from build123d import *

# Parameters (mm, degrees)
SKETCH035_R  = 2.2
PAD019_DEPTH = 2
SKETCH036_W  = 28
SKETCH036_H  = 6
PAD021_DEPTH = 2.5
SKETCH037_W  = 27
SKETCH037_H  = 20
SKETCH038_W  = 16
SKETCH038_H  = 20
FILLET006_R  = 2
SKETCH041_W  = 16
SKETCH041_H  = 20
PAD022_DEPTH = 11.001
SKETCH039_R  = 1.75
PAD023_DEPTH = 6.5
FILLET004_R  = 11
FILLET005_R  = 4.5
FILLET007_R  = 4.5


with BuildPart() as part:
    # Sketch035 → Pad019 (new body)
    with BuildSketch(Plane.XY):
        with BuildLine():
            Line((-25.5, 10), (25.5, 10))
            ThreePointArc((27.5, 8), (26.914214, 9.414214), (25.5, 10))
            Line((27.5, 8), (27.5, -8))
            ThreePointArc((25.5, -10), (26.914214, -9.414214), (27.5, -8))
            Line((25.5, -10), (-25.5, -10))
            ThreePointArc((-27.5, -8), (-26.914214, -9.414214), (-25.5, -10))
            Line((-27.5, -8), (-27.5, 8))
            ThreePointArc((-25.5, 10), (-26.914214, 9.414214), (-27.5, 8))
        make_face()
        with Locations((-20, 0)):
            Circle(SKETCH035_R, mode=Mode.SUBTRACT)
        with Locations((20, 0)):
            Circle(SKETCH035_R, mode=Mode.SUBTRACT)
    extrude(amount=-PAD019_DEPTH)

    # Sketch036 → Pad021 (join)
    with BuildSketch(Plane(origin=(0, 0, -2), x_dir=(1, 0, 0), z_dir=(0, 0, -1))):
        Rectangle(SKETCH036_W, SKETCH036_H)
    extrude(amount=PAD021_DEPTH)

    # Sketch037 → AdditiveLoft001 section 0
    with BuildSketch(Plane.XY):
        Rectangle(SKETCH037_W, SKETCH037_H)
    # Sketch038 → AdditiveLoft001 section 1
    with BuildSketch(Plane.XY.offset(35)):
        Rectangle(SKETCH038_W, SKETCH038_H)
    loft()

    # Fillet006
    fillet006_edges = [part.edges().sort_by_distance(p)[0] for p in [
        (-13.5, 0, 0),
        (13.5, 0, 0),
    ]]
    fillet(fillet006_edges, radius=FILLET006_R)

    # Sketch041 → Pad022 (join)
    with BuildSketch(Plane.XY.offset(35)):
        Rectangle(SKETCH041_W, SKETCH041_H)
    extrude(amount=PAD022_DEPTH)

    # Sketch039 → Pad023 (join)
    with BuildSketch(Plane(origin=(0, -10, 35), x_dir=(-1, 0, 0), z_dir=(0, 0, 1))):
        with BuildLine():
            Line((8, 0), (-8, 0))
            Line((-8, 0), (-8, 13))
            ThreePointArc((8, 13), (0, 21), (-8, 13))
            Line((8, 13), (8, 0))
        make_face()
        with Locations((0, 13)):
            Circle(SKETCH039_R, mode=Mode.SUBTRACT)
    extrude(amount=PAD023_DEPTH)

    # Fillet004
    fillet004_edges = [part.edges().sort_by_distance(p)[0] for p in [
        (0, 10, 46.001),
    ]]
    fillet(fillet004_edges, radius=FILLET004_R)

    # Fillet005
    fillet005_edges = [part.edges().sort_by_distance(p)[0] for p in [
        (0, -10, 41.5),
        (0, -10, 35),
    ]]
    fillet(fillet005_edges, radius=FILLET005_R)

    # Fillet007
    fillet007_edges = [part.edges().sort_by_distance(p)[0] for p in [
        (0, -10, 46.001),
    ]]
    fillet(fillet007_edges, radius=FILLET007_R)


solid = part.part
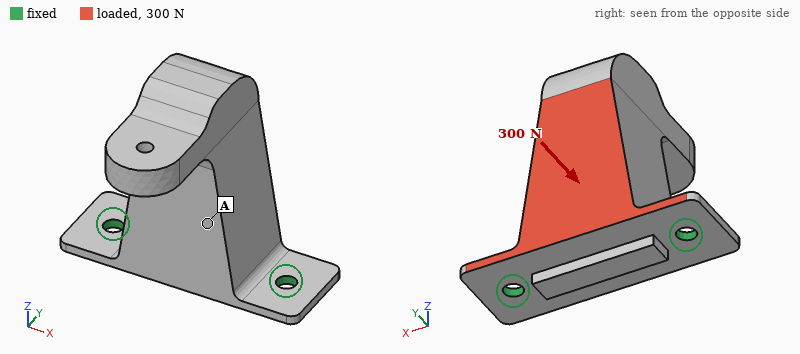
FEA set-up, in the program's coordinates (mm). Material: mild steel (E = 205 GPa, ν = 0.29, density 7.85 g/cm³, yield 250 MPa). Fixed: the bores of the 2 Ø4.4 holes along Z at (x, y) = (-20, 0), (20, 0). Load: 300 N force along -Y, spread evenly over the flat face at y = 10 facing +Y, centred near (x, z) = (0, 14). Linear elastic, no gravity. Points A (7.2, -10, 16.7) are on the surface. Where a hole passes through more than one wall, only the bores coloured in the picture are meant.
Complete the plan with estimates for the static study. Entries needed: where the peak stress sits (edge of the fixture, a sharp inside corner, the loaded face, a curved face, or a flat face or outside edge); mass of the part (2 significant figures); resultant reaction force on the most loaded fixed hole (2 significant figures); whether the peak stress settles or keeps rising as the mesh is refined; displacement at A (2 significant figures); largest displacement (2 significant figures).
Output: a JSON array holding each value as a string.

["edge of the fixture", "180 g", "150 N", "keeps rising", "37 µm", "96 µm"]
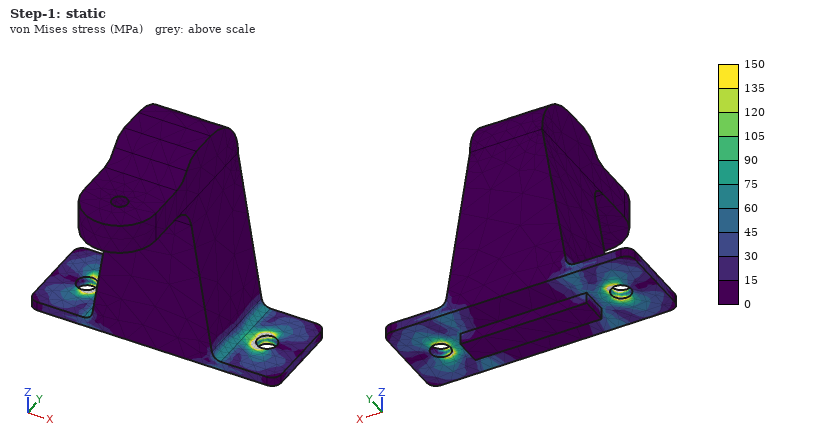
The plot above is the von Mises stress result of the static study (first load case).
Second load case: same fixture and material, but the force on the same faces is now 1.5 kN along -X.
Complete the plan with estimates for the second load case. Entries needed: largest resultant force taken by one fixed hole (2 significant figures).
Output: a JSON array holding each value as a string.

["1.1 kN"]
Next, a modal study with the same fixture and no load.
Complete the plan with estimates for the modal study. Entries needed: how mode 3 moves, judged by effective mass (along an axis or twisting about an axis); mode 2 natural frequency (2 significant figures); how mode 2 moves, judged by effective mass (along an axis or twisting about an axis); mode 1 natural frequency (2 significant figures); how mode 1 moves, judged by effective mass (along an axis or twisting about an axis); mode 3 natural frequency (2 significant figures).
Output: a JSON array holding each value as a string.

["along Z", "3000 Hz", "along X", "710 Hz", "along Y", "5000 Hz"]
